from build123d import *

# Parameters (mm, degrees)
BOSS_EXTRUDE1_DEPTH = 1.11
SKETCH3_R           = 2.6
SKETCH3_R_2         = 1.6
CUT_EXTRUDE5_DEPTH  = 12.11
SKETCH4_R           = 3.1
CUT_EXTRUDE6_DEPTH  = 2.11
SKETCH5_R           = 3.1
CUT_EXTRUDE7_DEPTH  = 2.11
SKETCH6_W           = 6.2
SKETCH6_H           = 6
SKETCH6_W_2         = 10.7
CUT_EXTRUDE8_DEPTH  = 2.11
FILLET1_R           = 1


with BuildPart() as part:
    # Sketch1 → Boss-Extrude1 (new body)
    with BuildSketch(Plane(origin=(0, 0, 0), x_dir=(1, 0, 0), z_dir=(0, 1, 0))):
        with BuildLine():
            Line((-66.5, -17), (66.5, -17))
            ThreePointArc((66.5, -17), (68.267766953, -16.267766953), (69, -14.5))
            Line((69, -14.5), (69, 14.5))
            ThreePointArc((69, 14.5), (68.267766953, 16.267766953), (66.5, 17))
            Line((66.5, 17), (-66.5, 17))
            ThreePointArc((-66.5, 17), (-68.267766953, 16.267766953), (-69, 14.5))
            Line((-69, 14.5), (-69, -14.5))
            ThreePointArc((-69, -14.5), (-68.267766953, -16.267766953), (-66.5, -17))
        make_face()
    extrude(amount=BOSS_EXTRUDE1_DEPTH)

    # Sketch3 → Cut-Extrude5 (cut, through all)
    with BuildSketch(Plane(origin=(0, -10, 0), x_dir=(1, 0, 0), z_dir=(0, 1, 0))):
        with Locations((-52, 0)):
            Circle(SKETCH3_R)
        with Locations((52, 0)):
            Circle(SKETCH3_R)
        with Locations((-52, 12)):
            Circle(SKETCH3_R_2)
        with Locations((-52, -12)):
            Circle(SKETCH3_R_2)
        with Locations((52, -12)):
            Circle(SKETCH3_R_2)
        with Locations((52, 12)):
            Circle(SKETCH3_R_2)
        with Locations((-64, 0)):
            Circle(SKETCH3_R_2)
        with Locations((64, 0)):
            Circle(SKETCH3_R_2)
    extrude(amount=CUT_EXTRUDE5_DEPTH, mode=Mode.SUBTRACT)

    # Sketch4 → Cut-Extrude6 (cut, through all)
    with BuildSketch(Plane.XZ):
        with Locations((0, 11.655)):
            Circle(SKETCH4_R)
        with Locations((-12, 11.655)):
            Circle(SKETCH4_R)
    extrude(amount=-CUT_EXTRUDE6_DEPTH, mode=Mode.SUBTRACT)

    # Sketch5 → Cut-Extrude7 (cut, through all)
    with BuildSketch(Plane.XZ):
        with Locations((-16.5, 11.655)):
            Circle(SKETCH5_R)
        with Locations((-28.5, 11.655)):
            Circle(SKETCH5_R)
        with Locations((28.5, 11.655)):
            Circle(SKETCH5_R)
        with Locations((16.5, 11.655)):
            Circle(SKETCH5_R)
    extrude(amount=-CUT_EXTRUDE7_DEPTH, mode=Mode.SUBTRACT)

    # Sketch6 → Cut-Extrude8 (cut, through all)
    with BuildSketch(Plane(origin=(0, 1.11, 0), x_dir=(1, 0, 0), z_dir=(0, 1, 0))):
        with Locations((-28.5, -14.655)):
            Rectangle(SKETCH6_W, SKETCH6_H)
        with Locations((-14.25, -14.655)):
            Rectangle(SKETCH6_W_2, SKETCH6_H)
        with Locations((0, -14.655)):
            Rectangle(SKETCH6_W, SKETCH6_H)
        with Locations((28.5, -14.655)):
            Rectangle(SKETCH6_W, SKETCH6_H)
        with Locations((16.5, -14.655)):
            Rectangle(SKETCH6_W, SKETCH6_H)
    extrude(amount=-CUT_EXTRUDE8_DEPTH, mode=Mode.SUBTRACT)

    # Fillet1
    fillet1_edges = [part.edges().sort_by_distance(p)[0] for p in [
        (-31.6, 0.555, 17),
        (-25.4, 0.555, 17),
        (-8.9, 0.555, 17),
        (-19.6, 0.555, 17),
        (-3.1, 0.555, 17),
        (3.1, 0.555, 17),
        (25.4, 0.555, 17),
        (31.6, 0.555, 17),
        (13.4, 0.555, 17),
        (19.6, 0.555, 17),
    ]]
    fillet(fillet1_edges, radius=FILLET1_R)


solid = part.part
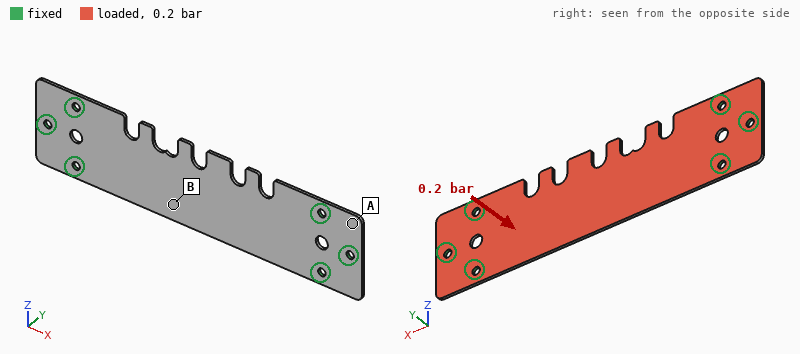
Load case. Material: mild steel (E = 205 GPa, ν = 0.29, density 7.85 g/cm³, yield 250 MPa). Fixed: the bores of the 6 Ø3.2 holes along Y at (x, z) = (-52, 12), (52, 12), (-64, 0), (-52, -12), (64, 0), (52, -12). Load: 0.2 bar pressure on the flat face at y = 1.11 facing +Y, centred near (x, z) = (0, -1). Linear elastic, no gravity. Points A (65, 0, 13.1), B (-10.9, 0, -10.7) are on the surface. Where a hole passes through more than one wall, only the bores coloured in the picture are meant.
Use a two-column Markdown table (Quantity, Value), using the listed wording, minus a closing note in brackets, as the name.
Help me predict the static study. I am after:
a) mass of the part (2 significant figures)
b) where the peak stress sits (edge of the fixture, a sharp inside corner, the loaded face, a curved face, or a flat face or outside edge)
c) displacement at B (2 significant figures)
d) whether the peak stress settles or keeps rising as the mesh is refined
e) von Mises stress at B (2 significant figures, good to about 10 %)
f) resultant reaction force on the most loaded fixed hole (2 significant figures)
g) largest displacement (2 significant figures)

| Quantity | Value |
|---|---|
| mass of the part | 38 g |
| where the peak stress sits | edge of the fixture |
| displacement at B | 0.23 mm |
| whether the peak stress settles or keeps rising as the mesh is refined | keeps rising |
| von Mises stress at B | 37 MPa |
| resultant reaction force on the most loaded fixed hole | 24 N |
| largest displacement | 0.27 mm |
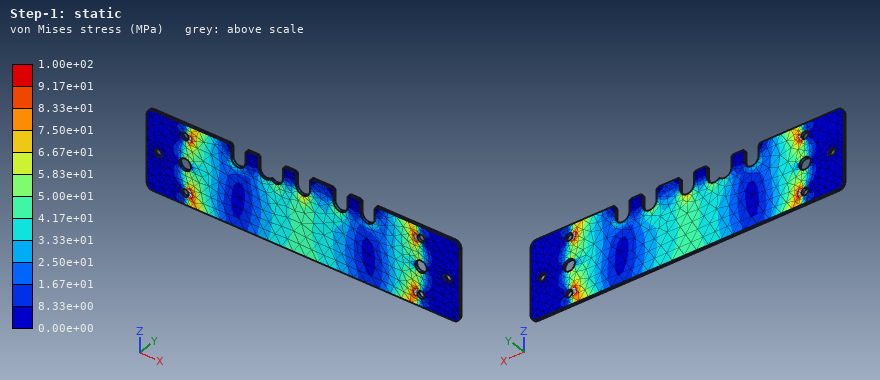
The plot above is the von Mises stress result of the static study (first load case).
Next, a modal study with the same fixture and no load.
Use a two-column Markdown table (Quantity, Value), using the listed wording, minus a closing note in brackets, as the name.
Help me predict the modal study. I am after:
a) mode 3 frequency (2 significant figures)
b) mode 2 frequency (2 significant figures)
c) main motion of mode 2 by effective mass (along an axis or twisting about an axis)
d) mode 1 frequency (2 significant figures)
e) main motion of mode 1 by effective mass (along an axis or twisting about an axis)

| Quantity | Value |
|---|---|
| mode 3 frequency | 1500 Hz |
| mode 2 frequency | 1300 Hz |
| main motion of mode 2 by effective mass | twisting about X |
| mode 1 frequency | 540 Hz |
| main motion of mode 1 by effective mass | along Y |
